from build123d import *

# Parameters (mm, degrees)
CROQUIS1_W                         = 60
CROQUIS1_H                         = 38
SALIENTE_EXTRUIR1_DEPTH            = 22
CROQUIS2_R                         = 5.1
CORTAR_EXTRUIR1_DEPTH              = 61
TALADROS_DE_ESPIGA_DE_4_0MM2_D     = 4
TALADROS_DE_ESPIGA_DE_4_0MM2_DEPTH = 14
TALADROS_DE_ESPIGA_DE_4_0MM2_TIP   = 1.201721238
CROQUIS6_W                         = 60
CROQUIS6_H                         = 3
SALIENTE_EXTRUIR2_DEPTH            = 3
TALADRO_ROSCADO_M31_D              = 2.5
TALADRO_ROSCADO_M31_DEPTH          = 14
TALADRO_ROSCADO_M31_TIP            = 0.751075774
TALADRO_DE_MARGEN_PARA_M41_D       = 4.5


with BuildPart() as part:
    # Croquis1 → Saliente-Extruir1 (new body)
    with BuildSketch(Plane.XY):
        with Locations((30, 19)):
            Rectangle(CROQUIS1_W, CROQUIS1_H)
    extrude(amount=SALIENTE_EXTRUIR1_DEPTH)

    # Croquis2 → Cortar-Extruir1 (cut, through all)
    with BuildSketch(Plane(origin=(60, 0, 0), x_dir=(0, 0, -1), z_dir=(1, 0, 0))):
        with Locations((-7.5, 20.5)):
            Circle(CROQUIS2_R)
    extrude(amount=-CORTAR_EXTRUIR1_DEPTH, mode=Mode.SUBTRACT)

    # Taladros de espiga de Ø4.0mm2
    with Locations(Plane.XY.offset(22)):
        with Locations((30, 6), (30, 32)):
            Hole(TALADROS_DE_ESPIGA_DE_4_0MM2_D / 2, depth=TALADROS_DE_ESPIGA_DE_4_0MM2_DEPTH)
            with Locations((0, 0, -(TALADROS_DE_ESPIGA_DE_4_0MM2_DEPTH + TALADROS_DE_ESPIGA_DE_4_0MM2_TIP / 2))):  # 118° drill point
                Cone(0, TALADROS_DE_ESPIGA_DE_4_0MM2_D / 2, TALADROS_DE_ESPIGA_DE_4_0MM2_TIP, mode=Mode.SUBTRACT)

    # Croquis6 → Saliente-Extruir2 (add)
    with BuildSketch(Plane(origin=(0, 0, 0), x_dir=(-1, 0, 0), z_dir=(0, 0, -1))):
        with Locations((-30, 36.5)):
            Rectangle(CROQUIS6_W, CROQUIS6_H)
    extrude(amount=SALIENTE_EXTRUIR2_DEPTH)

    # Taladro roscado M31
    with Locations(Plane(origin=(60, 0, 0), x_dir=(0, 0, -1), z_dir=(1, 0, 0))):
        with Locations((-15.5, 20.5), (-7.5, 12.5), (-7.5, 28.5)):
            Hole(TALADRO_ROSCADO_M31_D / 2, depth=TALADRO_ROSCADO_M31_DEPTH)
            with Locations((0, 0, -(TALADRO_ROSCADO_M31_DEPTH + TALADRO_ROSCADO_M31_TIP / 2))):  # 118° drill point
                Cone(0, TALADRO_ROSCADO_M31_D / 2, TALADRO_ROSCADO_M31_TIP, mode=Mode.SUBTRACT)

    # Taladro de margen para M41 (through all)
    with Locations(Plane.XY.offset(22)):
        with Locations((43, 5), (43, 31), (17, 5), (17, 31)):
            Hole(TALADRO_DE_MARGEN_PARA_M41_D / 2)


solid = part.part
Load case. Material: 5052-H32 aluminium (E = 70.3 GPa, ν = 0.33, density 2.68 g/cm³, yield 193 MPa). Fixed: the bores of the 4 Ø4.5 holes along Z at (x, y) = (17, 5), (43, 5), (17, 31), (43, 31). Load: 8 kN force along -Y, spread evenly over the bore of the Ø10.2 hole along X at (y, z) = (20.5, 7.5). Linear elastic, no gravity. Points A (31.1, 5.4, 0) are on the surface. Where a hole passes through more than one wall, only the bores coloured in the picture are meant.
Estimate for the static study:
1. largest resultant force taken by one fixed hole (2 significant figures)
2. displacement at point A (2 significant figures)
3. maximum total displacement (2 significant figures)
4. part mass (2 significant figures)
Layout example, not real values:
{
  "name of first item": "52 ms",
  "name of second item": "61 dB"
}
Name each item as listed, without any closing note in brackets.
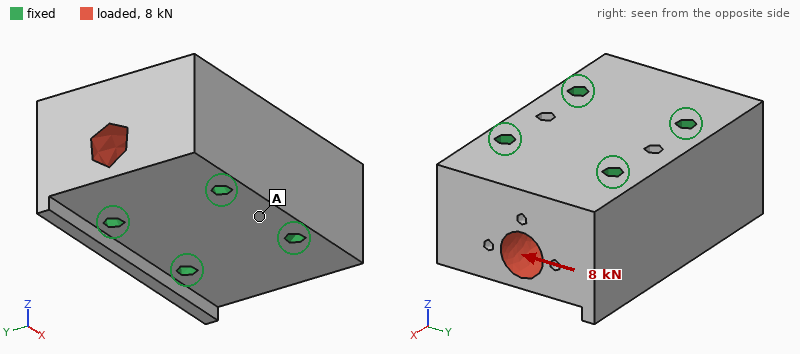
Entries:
{
  "largest resultant force taken by one fixed hole": "2.2 kN",
  "displacement at point A": "0.98 µm",
  "maximum total displacement": "2.8 µm",
  "part mass": "120 g"
}
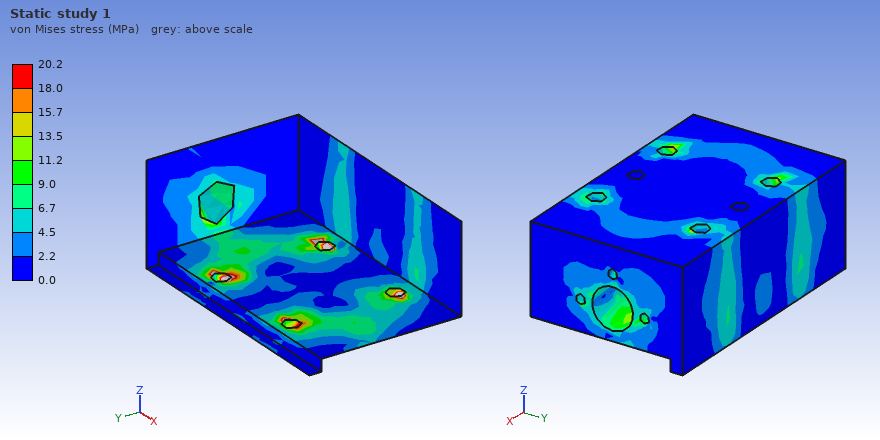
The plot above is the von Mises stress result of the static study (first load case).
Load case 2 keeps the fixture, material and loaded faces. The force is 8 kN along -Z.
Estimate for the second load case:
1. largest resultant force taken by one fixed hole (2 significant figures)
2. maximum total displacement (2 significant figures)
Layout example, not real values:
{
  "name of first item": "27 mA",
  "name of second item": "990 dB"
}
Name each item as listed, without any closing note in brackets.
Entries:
{
  "largest resultant force taken by one fixed hole": "2.3 kN",
  "maximum total displacement": "5.3 µm"
}
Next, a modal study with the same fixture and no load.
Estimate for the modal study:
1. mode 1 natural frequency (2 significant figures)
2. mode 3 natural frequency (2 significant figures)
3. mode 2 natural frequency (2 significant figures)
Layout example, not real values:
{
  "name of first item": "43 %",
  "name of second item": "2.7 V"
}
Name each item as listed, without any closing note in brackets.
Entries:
{
  "mode 1 natural frequency": "31 kHz",
  "mode 3 natural frequency": "36 kHz",
  "mode 2 natural frequency": "32 kHz"
}
